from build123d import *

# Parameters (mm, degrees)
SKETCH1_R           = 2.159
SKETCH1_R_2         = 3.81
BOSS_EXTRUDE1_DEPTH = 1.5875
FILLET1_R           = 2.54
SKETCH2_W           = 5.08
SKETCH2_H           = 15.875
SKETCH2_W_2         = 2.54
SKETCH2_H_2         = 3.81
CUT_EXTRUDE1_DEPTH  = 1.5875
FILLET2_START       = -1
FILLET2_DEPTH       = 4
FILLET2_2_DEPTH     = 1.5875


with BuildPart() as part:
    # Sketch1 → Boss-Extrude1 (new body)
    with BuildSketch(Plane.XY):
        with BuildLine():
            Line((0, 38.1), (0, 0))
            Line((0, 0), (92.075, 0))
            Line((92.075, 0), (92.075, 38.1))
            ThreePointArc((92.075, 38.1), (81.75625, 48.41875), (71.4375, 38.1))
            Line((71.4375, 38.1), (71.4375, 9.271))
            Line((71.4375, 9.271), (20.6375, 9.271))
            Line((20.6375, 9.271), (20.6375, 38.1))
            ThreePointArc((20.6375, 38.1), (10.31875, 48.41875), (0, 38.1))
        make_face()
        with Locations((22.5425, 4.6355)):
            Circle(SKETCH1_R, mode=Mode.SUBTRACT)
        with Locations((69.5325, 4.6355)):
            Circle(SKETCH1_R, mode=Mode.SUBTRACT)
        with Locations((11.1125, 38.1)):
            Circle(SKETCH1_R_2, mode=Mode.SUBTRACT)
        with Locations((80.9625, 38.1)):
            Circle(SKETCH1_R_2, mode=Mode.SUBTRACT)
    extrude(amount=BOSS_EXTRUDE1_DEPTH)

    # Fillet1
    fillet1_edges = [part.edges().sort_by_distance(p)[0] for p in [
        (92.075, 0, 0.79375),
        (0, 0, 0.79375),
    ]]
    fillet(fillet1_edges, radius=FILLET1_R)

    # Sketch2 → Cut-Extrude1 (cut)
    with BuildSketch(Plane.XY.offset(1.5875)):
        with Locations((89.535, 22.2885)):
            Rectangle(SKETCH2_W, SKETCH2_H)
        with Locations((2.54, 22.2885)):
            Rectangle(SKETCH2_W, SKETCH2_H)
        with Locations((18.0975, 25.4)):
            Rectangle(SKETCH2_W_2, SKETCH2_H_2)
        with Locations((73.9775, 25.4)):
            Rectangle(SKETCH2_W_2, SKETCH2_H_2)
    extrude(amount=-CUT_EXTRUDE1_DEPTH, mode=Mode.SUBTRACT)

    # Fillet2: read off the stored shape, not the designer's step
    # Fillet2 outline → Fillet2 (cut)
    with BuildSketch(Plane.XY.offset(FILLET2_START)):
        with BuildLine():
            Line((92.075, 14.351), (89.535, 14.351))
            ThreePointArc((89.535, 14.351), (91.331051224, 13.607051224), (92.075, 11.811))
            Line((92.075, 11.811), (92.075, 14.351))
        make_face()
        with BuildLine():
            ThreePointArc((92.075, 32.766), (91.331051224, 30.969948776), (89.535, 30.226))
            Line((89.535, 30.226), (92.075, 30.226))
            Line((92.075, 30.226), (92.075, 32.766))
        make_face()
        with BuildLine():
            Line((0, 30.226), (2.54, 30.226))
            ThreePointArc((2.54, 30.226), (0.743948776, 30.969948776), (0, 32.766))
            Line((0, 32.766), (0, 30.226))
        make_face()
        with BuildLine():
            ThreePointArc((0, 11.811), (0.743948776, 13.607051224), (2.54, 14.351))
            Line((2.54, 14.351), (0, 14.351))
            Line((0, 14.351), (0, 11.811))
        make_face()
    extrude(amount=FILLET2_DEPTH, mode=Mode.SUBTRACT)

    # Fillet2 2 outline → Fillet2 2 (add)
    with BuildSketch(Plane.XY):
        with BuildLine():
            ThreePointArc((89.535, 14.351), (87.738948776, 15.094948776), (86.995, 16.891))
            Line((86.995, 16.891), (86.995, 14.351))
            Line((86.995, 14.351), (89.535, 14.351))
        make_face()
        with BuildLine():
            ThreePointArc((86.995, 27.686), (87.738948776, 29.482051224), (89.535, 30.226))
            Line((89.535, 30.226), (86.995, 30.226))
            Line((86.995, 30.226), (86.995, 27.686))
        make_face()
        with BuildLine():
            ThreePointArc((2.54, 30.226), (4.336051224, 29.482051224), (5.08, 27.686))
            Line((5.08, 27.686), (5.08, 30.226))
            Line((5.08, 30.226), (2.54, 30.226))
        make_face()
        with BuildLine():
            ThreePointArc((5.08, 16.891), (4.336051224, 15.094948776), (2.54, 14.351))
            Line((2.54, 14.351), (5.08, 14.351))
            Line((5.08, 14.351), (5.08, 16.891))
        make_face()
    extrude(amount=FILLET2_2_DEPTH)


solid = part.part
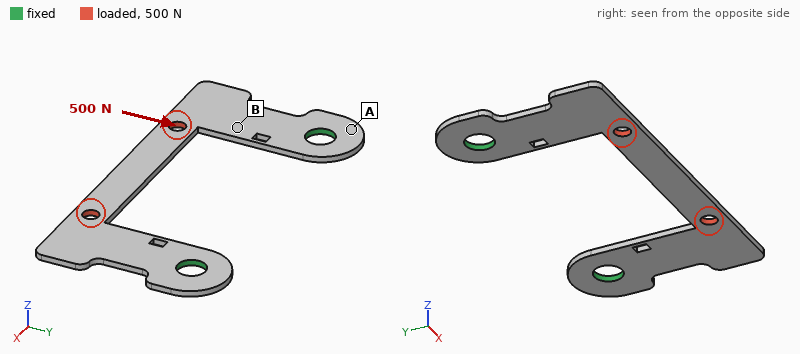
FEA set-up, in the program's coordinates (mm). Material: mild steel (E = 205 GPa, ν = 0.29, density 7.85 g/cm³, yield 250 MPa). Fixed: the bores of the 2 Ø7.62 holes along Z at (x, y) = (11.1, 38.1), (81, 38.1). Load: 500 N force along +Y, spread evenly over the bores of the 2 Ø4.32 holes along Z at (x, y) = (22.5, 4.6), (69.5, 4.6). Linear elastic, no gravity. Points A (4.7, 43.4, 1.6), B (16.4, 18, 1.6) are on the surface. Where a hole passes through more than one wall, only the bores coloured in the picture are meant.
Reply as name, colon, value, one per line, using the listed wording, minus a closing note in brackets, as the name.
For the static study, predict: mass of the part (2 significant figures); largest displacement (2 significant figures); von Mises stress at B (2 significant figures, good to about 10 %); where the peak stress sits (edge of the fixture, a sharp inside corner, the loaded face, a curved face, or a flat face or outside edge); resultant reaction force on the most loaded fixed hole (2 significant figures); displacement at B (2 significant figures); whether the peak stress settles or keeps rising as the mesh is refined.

mass of the part: 26 g
largest displacement: 9.4 µm
von Mises stress at B: 20 MPa
where the peak stress sits: a sharp inside corner
resultant reaction force on the most loaded fixed hole: 270 N
displacement at B: 1.4 µm
whether the peak stress settles or keeps rising as the mesh is refined: keeps rising
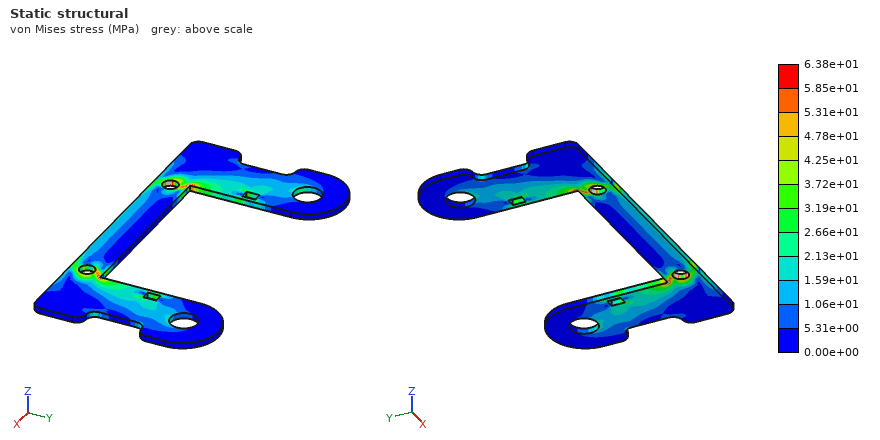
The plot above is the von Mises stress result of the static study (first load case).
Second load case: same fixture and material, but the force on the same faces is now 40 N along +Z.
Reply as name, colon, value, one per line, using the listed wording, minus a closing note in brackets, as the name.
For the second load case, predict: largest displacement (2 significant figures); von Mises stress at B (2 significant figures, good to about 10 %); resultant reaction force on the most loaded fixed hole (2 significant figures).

largest displacement: 0.27 mm
von Mises stress at B: 42 MPa
resultant reaction force on the most loaded fixed hole: 20 N
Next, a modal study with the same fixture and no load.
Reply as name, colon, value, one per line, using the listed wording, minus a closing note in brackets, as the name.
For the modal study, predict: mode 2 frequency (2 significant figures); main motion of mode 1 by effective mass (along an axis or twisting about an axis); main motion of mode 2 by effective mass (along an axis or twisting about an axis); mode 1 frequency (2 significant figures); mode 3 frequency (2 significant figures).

mode 2 frequency: 1100 Hz
main motion of mode 1 by effective mass: along Z
main motion of mode 2 by effective mass: twisting about Y
mode 1 frequency: 660 Hz
mode 3 frequency: 1700 Hz
